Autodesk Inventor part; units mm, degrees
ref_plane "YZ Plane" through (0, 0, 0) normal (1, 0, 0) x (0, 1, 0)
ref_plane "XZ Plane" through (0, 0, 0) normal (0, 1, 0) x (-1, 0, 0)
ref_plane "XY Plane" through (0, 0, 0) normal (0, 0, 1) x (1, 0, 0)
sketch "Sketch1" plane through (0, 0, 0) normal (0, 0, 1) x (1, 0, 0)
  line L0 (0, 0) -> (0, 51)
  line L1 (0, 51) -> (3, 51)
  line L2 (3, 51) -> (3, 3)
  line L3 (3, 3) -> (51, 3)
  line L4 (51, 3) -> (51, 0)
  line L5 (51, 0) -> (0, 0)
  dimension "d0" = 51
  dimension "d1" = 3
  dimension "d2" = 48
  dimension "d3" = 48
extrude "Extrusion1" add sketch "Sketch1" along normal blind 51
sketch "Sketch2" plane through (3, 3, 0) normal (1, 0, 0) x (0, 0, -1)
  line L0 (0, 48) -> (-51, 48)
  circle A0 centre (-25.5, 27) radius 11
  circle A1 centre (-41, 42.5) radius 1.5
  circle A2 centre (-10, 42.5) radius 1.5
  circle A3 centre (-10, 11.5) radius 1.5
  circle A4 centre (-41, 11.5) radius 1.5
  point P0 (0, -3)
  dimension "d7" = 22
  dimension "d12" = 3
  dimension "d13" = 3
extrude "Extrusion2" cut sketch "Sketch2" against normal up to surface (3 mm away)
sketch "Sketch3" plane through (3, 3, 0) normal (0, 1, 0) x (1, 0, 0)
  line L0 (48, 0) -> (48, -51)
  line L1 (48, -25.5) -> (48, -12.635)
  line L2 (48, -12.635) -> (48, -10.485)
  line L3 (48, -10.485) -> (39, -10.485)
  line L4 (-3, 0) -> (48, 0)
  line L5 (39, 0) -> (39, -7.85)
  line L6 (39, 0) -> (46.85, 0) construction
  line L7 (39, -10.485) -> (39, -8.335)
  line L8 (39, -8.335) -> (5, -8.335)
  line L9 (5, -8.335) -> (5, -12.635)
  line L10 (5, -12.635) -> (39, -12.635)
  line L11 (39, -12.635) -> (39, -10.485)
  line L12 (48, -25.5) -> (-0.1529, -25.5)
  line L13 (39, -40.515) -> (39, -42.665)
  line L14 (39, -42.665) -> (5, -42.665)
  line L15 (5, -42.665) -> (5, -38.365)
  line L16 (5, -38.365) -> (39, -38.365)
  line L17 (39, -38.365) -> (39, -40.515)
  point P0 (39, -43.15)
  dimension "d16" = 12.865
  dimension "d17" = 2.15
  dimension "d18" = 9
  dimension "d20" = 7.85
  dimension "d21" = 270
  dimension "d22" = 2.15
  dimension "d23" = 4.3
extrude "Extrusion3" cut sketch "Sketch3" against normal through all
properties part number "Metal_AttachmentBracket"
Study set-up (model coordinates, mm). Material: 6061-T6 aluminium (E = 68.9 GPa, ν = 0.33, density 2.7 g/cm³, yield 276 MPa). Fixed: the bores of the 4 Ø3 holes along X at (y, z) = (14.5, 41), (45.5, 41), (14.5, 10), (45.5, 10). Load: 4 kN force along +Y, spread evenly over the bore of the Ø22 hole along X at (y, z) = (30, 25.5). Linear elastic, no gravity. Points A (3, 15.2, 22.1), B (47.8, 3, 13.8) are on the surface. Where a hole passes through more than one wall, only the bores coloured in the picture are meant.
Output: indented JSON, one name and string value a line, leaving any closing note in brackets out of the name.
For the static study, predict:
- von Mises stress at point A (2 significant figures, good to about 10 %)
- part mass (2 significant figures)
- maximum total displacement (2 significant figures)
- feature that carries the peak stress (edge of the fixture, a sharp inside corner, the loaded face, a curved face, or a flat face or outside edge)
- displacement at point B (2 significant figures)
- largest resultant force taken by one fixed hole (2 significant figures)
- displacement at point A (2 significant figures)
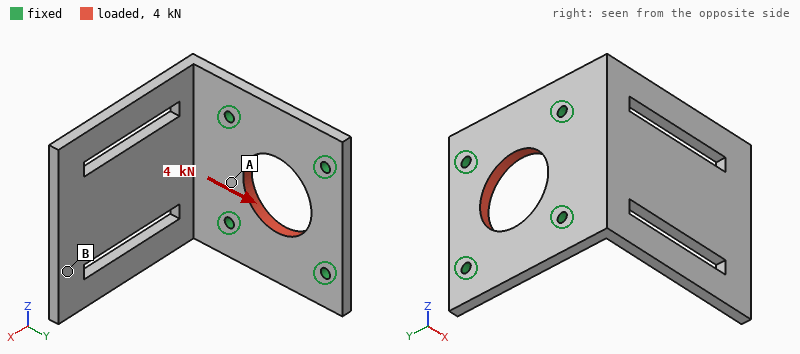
{
  "von Mises stress at point A": "15 MPa",
  "part mass": "35 g",
  "maximum total displacement": "13 µm",
  "feature that carries the peak stress": "edge of the fixture",
  "displacement at point B": "4.4 µm",
  "largest resultant force taken by one fixed hole": "1.0 kN",
  "displacement at point A": "6.0 µm"
}
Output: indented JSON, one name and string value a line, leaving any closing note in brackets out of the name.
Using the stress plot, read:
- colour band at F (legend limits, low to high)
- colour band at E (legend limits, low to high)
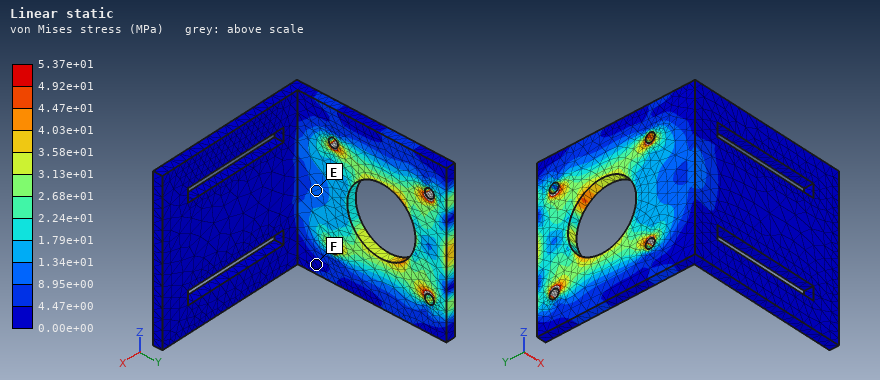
{
  "colour band at F": "0.00e+00 to 4.47e+00 MPa",
  "colour band at E": "8.95e+00 to 1.34e+01 MPa"
}
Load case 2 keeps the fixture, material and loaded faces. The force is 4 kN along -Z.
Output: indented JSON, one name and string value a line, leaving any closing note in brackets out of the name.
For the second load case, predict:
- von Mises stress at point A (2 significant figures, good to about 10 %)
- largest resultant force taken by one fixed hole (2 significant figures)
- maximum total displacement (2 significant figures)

{
  "von Mises stress at point A": "22 MPa",
  "largest resultant force taken by one fixed hole": "1.0 kN",
  "maximum total displacement": "9.3 µm"
}
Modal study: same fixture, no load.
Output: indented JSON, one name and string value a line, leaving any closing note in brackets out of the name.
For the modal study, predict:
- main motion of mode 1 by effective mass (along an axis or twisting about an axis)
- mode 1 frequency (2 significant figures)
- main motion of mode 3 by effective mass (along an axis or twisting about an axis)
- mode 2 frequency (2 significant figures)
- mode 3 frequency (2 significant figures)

{
  "main motion of mode 1 by effective mass": "along Y",
  "mode 1 frequency": "710 Hz",
  "main motion of mode 3 by effective mass": "along Z",
  "mode 2 frequency": "1800 Hz",
  "mode 3 frequency": "2500 Hz"
}
